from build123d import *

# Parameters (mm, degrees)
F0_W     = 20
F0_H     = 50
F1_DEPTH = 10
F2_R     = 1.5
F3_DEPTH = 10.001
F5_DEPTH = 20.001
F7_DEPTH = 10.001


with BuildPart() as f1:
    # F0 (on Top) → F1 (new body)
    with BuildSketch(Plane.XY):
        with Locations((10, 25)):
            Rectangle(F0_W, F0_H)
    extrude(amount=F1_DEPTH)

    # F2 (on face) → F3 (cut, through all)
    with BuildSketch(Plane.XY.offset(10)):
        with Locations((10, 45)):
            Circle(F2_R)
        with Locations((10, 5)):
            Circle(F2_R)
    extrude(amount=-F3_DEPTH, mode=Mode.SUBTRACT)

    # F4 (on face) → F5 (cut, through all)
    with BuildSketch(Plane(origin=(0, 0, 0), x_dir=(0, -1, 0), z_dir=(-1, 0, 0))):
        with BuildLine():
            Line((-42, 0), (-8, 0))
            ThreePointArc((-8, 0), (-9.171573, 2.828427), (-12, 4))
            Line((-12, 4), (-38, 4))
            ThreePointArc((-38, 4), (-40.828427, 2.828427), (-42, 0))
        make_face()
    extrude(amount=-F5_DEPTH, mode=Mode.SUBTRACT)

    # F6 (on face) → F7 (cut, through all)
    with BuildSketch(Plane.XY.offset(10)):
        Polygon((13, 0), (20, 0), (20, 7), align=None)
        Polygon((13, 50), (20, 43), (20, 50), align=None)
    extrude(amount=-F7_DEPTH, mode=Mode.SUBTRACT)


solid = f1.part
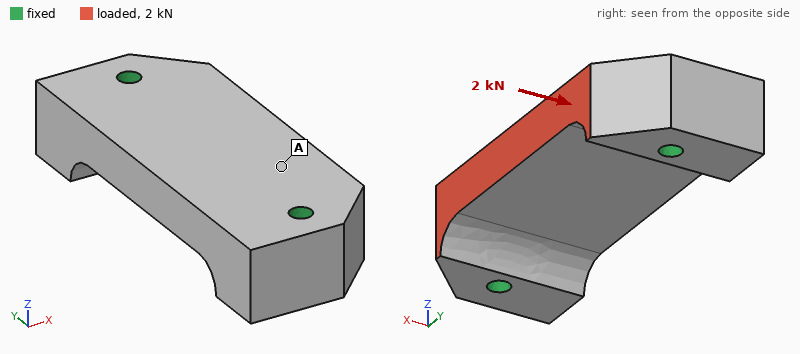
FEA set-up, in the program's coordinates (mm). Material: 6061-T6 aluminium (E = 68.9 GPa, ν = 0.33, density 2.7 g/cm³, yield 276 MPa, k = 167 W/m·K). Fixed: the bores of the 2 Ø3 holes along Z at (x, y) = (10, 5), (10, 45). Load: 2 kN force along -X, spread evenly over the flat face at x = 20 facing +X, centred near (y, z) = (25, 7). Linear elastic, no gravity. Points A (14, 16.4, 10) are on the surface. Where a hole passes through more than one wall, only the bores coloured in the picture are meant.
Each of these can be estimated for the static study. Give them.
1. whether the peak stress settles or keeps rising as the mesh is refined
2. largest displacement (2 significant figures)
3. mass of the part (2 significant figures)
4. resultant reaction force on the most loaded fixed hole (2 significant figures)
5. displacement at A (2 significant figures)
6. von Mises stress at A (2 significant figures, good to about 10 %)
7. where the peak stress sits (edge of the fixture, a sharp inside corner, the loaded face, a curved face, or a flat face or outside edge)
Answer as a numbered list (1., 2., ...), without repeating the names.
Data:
1. keeps rising
2. 8.9 µm
3. 18 g
4. 1.0 kN
5. 6.8 µm
6. 11 MPa
7. edge of the fixture
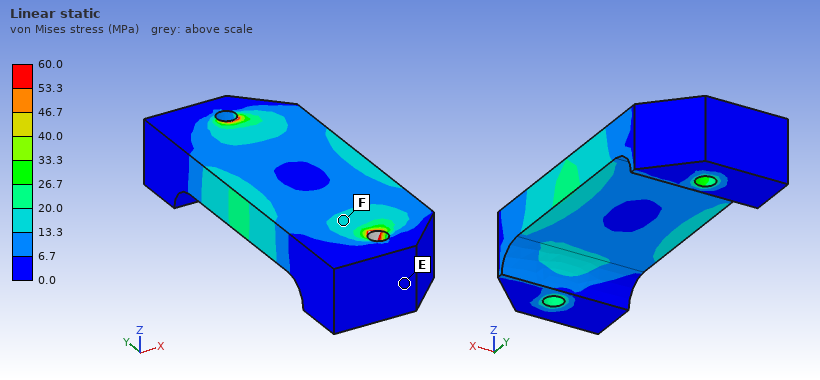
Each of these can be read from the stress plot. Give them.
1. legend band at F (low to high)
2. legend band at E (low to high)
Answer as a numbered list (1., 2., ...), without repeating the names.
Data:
1. 13.3 to 20.0 MPa
2. 0.0 to 6.7 MPa
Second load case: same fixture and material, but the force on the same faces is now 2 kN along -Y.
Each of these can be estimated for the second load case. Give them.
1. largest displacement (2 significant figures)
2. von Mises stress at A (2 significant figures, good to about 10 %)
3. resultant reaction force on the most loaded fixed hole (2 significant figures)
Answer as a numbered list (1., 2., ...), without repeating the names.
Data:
1. 4.4 µm
2. 11 MPa
3. 1.1 kN
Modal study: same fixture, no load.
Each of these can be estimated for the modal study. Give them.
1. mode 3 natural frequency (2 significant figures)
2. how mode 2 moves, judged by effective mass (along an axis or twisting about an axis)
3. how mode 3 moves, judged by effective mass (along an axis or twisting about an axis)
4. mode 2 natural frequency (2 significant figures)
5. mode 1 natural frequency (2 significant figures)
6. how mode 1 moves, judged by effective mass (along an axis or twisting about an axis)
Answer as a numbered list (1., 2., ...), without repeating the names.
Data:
1. 25 kHz
2. along X
3. along X
4. 23 kHz
5. 19 kHz
6. along Z
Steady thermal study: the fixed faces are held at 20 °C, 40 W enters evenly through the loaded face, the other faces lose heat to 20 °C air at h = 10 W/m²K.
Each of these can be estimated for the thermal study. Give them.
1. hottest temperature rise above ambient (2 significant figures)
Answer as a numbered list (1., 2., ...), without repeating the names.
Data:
1. 18 K
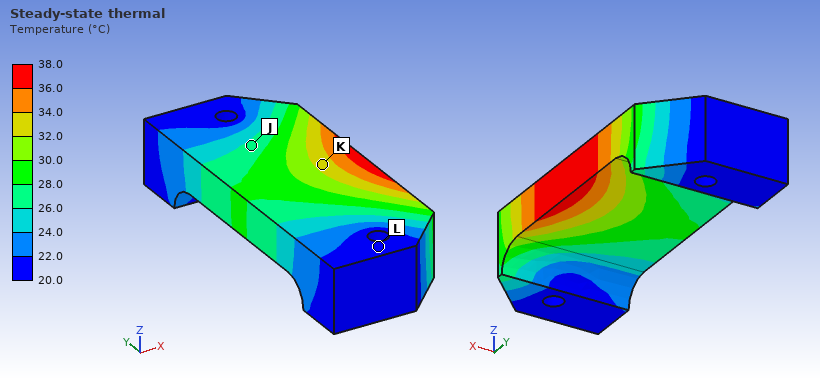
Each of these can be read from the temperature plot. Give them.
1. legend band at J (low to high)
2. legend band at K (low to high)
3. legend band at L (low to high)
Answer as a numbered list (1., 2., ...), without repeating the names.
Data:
1. 26.0 to 28.0 °C
2. 32.0 to 34.0 °C
3. 20.0 to 22.0 °C
